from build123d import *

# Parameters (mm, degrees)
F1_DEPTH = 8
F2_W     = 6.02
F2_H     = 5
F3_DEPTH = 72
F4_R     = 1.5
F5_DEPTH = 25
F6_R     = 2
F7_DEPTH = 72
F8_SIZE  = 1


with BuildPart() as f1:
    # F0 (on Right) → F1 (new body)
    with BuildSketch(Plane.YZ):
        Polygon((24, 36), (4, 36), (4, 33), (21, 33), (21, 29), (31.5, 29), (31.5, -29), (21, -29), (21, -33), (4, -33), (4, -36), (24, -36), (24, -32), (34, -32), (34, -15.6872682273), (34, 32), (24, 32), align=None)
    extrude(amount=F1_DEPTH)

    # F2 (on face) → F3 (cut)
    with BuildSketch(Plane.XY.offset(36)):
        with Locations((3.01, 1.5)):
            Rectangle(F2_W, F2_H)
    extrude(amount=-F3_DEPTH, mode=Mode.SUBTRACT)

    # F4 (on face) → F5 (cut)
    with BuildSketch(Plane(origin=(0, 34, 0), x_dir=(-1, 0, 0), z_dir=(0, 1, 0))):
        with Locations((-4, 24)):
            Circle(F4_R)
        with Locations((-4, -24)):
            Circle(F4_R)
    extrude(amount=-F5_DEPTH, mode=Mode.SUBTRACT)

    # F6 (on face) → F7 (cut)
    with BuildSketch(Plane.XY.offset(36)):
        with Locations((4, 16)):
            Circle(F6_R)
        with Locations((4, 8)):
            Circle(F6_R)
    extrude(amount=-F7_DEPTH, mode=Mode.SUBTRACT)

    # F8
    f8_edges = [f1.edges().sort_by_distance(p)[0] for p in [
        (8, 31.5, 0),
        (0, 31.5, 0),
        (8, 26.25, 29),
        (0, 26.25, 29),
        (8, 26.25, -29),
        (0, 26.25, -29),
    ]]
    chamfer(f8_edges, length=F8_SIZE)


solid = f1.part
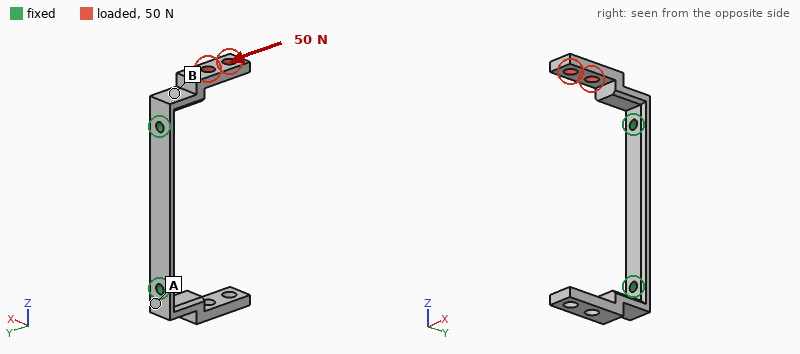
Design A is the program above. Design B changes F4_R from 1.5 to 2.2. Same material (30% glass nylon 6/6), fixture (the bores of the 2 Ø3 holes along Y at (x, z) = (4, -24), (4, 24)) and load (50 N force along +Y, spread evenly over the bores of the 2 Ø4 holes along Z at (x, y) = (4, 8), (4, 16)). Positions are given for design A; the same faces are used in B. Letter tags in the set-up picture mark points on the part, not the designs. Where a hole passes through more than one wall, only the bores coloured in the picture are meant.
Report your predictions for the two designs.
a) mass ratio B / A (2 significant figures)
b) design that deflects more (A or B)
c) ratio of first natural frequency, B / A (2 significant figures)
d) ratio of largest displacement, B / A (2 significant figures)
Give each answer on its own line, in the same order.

0.98
A
1.1
0.86
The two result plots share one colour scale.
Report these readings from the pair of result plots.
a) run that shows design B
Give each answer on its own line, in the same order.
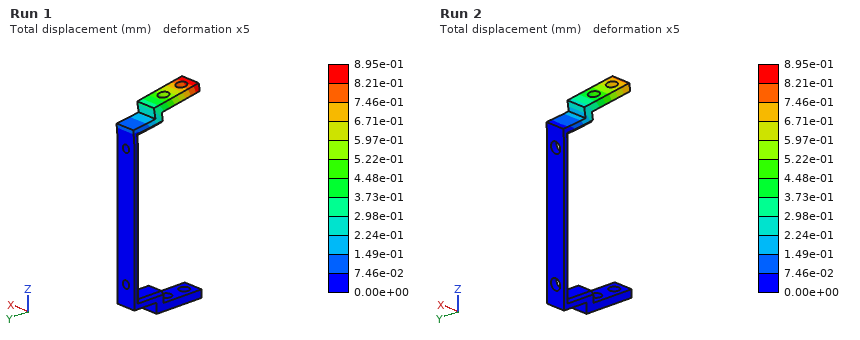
Run 2
